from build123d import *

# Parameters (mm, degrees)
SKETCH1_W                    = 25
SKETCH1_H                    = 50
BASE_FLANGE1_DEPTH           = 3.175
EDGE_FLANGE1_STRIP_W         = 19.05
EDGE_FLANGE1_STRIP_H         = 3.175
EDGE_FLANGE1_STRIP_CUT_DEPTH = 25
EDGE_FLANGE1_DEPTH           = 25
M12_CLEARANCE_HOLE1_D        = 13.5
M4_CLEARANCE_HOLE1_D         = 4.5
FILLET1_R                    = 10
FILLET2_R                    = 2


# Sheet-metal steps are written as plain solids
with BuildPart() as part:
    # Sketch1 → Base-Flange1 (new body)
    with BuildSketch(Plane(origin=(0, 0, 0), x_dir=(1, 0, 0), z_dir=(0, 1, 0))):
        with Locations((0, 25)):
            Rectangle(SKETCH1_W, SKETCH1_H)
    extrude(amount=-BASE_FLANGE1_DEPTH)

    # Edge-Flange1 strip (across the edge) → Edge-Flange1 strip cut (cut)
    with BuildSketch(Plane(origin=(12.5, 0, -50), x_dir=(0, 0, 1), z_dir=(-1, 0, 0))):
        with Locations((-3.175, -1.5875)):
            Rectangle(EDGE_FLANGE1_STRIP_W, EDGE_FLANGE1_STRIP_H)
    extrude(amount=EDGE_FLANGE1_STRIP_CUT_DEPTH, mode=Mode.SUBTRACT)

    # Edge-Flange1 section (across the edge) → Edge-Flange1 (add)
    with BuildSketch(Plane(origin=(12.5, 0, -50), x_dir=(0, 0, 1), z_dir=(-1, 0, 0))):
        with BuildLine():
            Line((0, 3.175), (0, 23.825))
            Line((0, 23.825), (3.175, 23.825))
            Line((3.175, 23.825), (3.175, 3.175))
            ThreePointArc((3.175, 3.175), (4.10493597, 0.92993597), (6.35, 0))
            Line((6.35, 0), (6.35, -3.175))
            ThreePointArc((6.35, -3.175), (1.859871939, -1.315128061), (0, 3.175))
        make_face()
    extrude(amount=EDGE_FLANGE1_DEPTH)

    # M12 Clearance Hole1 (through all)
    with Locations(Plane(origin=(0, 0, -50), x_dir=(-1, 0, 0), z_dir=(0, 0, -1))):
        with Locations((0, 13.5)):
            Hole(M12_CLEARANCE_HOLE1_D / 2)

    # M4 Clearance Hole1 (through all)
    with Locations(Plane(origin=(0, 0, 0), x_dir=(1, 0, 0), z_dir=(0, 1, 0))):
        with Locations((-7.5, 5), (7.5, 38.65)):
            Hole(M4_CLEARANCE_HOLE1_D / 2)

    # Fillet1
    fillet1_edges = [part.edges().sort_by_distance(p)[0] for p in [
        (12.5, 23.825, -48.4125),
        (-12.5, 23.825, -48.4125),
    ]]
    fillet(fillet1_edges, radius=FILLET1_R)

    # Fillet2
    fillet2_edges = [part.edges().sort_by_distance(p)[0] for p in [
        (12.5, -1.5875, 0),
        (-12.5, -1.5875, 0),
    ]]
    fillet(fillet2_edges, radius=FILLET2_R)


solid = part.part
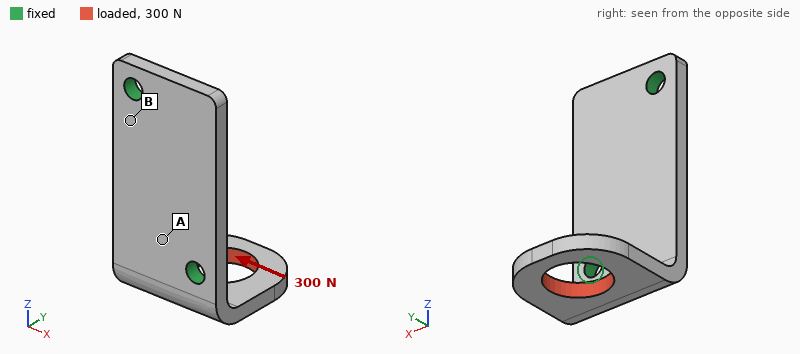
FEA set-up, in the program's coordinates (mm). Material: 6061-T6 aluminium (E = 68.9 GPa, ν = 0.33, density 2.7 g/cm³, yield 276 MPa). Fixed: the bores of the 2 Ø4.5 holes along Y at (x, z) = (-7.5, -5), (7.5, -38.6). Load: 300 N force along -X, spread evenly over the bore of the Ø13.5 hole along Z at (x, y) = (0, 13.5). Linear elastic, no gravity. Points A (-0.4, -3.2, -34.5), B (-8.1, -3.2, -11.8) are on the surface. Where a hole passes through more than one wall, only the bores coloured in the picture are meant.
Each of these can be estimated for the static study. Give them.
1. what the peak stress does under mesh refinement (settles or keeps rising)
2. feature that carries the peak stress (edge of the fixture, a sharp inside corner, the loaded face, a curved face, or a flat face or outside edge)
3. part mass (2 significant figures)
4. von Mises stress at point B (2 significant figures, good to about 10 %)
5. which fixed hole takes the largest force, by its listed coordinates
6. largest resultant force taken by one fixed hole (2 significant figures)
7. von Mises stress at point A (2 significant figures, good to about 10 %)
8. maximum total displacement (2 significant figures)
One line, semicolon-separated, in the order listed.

keeps rising; edge of the fixture; 14 g; 18 MPa; (7.5, -38.6); 330 N; 41 MPa; 0.18 mm
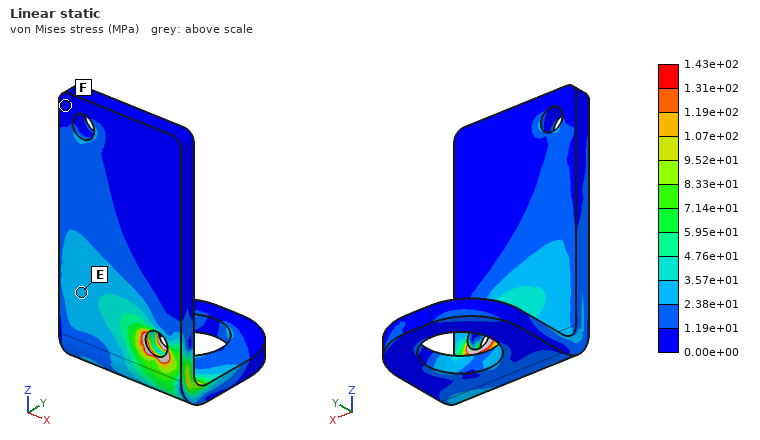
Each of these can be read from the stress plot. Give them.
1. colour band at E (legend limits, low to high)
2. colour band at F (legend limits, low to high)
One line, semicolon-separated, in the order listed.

2.38e+01 to 3.57e+01 MPa; 0.00e+00 to 1.19e+01 MPa
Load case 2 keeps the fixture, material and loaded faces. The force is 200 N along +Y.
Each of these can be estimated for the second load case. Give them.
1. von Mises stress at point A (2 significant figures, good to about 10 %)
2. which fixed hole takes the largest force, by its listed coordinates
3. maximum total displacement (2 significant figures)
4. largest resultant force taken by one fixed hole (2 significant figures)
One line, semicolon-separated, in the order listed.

19 MPa; (7.5, -38.6); 90 µm; 210 N
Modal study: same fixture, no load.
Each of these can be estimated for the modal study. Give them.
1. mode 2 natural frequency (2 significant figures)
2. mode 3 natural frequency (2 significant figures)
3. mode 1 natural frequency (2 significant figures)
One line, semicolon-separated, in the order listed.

4100 Hz; 8000 Hz; 3100 Hz
